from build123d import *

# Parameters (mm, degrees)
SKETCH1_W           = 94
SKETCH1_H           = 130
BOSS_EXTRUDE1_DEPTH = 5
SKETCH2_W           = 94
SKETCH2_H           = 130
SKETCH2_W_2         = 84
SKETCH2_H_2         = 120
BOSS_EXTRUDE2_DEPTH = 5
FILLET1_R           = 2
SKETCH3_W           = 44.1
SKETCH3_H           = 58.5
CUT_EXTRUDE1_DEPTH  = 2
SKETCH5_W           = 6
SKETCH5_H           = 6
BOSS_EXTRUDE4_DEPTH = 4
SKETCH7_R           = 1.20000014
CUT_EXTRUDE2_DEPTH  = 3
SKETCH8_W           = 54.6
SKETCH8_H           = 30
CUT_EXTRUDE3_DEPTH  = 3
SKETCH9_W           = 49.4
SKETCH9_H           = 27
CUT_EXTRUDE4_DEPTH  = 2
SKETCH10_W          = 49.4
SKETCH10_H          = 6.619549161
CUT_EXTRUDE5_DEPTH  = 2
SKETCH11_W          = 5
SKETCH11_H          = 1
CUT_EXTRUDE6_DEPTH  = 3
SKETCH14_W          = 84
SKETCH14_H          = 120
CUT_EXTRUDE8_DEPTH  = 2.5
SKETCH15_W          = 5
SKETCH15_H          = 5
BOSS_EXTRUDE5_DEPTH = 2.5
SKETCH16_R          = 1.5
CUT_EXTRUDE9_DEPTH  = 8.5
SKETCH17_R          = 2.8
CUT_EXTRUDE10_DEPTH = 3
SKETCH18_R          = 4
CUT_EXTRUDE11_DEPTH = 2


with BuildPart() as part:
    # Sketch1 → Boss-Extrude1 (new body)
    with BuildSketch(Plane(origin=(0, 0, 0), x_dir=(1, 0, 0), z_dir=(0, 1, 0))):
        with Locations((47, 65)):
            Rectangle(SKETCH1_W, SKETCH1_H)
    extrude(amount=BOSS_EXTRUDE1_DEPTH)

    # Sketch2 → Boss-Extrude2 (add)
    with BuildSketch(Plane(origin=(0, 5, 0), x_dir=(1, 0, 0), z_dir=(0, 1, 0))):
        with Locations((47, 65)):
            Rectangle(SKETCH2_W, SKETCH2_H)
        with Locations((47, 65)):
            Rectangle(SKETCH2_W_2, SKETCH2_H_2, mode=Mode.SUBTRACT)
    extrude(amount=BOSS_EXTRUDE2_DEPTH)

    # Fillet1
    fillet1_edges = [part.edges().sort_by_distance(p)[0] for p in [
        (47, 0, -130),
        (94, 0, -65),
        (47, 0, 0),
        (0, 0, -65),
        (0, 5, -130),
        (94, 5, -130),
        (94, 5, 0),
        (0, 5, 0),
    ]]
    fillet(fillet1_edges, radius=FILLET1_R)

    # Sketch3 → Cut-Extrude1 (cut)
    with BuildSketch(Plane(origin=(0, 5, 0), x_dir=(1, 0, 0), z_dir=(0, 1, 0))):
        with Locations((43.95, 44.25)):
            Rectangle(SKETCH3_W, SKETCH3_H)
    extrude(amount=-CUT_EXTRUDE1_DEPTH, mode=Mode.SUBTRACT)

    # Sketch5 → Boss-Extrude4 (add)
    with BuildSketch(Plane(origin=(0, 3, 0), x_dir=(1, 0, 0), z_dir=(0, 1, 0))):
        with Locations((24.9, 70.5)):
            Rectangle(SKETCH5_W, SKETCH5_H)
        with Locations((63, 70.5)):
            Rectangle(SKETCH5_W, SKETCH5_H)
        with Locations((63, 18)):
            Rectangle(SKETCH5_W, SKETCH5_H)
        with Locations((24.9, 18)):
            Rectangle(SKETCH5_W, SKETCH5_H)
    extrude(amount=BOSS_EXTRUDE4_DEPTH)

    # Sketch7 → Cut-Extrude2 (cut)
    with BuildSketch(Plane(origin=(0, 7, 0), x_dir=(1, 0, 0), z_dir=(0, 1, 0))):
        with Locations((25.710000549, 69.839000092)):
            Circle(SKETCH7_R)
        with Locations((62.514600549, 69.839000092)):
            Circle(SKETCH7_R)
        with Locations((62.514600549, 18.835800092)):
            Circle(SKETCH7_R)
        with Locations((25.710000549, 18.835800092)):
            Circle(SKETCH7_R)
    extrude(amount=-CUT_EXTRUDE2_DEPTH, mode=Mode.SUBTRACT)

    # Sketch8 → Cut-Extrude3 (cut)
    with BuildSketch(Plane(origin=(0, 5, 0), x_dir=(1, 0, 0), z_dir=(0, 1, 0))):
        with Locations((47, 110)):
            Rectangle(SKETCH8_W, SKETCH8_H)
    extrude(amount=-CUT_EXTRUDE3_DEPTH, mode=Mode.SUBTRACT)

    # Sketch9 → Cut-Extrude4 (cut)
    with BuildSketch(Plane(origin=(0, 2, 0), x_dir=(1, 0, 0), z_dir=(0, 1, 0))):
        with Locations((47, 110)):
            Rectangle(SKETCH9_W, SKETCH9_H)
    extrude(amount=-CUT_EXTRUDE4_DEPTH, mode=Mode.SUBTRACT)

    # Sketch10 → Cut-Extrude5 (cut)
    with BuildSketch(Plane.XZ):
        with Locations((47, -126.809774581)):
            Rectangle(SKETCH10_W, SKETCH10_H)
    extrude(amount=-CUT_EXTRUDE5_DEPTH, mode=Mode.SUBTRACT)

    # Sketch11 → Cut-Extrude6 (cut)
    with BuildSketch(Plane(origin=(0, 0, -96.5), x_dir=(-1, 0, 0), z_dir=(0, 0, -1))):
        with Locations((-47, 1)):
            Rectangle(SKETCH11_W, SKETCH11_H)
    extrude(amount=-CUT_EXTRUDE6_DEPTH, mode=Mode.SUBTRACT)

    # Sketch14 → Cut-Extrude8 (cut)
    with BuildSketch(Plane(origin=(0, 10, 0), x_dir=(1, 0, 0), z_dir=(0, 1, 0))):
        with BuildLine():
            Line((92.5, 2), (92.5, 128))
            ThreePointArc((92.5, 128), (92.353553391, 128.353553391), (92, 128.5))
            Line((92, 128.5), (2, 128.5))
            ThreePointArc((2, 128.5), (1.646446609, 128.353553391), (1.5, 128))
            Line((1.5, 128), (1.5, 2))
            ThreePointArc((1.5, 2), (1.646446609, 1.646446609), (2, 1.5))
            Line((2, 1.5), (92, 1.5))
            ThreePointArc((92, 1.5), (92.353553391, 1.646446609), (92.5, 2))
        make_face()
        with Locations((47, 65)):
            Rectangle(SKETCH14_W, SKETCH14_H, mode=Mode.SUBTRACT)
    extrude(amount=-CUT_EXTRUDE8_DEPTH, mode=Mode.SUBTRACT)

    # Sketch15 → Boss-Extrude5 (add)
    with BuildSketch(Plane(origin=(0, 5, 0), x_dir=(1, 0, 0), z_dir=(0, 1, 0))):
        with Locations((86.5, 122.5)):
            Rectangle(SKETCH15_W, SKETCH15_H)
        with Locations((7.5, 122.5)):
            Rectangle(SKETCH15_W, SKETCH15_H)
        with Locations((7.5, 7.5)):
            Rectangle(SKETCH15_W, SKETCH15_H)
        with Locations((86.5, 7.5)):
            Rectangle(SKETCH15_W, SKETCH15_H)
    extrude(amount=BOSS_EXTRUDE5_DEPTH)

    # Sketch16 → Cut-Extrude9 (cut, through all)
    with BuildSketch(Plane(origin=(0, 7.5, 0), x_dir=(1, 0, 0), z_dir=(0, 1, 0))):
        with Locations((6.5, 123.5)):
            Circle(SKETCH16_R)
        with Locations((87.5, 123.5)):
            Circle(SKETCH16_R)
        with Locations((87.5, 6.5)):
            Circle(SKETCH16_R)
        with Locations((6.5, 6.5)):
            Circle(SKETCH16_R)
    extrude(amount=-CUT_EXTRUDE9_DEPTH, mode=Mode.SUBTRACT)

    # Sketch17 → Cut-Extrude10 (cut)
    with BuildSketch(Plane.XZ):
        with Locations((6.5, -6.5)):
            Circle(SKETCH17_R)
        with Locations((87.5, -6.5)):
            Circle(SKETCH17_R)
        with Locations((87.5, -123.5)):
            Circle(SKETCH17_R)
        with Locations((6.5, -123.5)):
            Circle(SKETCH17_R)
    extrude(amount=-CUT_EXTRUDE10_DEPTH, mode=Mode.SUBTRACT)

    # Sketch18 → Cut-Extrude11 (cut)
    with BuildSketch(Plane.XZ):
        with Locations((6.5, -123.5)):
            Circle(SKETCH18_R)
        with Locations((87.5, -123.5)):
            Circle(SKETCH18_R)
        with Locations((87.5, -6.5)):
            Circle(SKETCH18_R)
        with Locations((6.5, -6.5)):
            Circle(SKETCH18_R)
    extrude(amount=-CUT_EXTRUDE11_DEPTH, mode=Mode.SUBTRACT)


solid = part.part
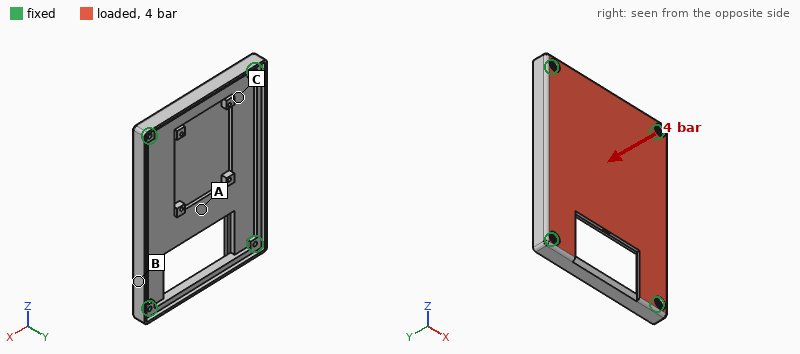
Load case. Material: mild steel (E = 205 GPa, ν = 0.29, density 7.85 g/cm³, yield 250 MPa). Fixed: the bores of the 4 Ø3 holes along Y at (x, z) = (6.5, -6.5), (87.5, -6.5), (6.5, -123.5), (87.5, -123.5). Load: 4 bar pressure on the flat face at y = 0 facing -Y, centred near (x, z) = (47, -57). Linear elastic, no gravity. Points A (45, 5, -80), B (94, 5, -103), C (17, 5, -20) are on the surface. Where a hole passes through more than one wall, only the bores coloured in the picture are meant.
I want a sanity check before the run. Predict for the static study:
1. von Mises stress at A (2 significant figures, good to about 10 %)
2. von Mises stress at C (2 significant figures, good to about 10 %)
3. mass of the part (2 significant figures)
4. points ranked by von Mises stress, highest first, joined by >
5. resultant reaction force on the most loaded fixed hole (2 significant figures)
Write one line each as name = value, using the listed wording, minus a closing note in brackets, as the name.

von Mises stress at A = 61 MPa
von Mises stress at C = 38 MPa
mass of the part = 430 g
points ranked by von Mises stress, highest first, joined by > = A > C > B
resultant reaction force on the most loaded fixed hole = 2.5 kN
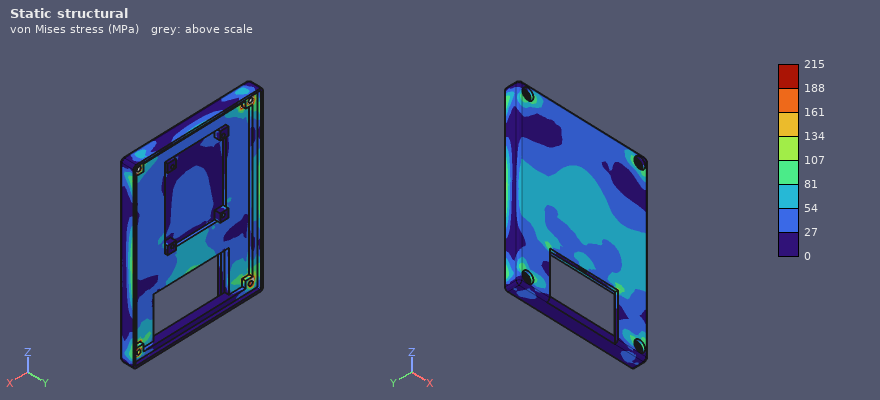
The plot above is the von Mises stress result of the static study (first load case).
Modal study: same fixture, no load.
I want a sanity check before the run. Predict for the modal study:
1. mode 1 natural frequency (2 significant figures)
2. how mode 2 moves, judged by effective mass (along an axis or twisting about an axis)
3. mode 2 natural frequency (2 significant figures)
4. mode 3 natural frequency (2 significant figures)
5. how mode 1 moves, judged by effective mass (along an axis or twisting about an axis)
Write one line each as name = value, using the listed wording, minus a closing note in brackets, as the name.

mode 1 natural frequency = 1600 Hz
how mode 2 moves, judged by effective mass = twisting about Z
mode 2 natural frequency = 2300 Hz
mode 3 natural frequency = 3500 Hz
how mode 1 moves, judged by effective mass = along Y
